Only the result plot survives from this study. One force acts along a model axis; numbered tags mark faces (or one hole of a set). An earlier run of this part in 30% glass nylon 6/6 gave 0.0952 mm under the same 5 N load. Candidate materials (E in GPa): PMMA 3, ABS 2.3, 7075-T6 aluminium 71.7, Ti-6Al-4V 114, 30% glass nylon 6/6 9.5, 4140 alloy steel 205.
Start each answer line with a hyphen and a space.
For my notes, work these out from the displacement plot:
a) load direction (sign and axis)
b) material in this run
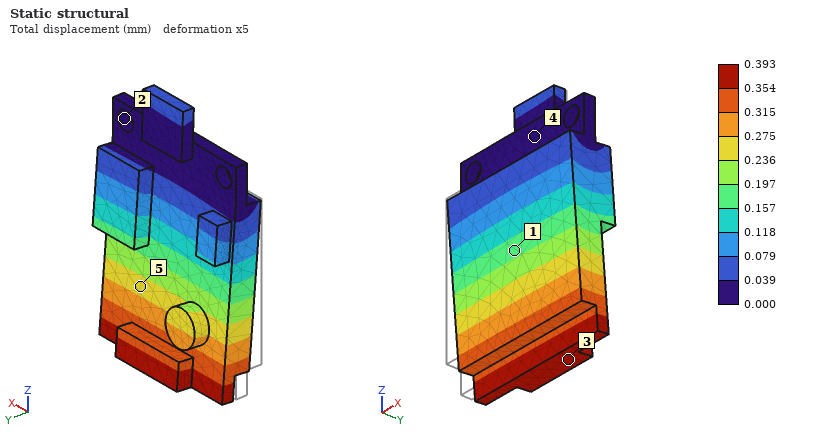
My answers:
- +Y
- ABS
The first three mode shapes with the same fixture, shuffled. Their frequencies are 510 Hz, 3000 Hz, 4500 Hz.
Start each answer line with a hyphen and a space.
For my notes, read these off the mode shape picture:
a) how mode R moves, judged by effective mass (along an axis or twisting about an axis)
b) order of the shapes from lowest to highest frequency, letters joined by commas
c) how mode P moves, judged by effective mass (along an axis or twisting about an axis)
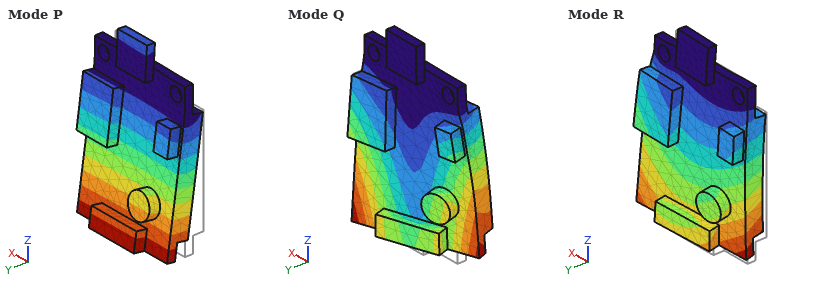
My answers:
- along X
- P, Q, R
- along Y
